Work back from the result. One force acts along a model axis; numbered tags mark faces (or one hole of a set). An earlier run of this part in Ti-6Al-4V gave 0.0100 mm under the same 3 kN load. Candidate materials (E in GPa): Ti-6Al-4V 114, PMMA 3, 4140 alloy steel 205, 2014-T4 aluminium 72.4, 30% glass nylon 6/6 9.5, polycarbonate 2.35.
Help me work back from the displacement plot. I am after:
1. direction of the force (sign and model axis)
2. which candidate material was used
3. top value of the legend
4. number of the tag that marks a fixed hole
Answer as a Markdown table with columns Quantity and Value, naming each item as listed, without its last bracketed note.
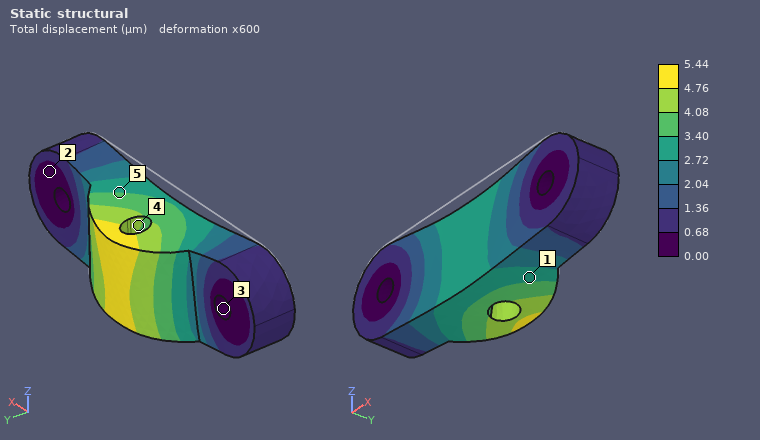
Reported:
| Quantity | Value |
|---|---|
| direction of the force | -Z |
| which candidate material was used | 4140 alloy steel |
| top value of the legend | 5.44 µm |
| number of the tag that marks a fixed hole | 3 |
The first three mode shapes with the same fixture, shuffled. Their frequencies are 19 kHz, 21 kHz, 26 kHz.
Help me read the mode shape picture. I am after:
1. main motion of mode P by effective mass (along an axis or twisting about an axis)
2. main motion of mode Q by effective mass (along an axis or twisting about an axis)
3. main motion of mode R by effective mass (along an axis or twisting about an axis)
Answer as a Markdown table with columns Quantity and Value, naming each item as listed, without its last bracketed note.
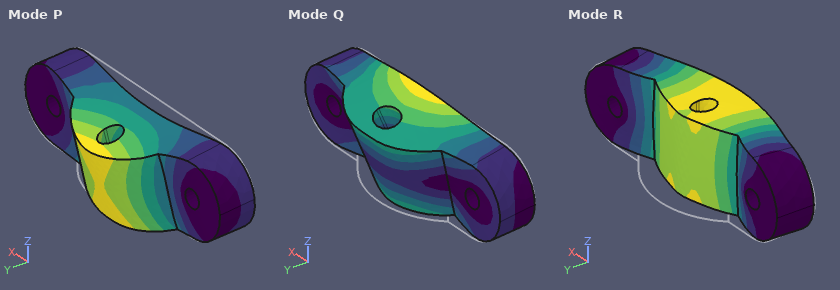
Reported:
| Quantity | Value |
|---|---|
| main motion of mode P by effective mass | along Z |
| main motion of mode Q by effective mass | along Z |
| main motion of mode R by effective mass | along Y |
